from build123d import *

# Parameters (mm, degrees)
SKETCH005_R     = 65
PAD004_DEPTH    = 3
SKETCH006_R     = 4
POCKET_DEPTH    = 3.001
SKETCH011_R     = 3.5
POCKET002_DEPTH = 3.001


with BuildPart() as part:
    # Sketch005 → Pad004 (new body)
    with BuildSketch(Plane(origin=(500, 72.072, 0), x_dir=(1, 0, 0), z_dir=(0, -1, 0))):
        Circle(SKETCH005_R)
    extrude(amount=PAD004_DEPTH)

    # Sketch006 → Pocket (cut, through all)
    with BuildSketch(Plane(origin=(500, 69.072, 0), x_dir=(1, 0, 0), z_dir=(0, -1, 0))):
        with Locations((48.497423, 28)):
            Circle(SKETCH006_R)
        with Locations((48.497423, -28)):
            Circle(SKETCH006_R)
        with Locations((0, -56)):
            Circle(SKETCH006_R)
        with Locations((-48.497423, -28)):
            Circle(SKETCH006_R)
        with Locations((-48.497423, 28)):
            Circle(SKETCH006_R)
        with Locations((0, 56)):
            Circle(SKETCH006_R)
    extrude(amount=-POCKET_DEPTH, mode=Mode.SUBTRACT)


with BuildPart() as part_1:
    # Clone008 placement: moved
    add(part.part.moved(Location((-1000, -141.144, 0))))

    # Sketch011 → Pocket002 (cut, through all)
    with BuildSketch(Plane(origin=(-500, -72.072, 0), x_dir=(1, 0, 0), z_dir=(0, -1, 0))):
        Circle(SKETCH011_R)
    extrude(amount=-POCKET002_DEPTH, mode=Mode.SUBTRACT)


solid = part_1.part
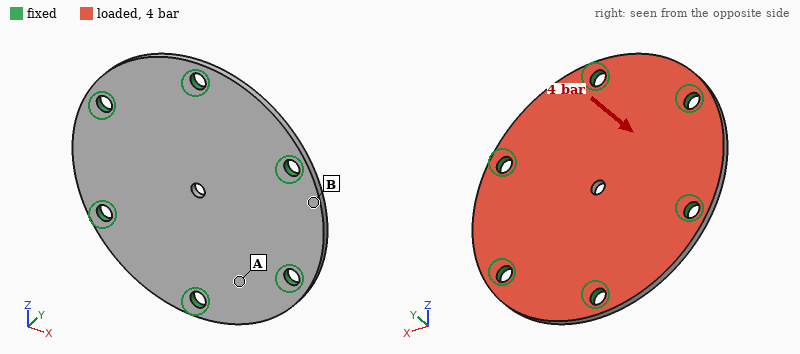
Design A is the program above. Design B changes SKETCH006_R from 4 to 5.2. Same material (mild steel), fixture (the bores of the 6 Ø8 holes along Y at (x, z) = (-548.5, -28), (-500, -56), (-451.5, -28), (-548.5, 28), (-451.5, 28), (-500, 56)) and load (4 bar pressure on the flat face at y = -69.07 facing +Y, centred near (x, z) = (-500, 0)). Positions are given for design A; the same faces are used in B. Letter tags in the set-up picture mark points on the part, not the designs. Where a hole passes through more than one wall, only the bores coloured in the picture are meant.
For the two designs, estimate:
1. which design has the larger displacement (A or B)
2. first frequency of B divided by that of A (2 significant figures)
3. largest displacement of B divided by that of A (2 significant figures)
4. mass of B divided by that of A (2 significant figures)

A
1.1
0.89
0.98
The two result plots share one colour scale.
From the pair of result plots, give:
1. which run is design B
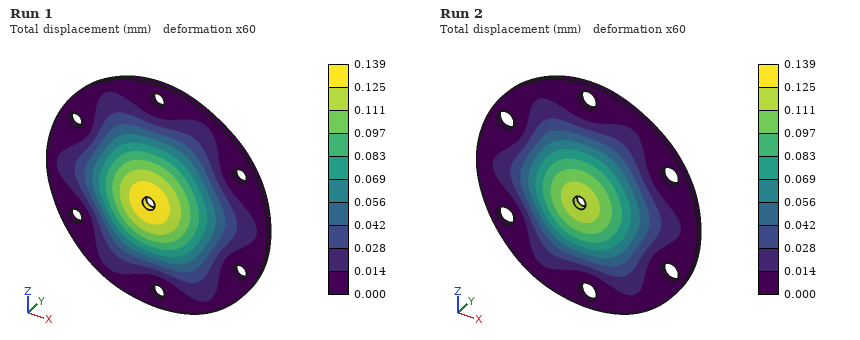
Run 2
